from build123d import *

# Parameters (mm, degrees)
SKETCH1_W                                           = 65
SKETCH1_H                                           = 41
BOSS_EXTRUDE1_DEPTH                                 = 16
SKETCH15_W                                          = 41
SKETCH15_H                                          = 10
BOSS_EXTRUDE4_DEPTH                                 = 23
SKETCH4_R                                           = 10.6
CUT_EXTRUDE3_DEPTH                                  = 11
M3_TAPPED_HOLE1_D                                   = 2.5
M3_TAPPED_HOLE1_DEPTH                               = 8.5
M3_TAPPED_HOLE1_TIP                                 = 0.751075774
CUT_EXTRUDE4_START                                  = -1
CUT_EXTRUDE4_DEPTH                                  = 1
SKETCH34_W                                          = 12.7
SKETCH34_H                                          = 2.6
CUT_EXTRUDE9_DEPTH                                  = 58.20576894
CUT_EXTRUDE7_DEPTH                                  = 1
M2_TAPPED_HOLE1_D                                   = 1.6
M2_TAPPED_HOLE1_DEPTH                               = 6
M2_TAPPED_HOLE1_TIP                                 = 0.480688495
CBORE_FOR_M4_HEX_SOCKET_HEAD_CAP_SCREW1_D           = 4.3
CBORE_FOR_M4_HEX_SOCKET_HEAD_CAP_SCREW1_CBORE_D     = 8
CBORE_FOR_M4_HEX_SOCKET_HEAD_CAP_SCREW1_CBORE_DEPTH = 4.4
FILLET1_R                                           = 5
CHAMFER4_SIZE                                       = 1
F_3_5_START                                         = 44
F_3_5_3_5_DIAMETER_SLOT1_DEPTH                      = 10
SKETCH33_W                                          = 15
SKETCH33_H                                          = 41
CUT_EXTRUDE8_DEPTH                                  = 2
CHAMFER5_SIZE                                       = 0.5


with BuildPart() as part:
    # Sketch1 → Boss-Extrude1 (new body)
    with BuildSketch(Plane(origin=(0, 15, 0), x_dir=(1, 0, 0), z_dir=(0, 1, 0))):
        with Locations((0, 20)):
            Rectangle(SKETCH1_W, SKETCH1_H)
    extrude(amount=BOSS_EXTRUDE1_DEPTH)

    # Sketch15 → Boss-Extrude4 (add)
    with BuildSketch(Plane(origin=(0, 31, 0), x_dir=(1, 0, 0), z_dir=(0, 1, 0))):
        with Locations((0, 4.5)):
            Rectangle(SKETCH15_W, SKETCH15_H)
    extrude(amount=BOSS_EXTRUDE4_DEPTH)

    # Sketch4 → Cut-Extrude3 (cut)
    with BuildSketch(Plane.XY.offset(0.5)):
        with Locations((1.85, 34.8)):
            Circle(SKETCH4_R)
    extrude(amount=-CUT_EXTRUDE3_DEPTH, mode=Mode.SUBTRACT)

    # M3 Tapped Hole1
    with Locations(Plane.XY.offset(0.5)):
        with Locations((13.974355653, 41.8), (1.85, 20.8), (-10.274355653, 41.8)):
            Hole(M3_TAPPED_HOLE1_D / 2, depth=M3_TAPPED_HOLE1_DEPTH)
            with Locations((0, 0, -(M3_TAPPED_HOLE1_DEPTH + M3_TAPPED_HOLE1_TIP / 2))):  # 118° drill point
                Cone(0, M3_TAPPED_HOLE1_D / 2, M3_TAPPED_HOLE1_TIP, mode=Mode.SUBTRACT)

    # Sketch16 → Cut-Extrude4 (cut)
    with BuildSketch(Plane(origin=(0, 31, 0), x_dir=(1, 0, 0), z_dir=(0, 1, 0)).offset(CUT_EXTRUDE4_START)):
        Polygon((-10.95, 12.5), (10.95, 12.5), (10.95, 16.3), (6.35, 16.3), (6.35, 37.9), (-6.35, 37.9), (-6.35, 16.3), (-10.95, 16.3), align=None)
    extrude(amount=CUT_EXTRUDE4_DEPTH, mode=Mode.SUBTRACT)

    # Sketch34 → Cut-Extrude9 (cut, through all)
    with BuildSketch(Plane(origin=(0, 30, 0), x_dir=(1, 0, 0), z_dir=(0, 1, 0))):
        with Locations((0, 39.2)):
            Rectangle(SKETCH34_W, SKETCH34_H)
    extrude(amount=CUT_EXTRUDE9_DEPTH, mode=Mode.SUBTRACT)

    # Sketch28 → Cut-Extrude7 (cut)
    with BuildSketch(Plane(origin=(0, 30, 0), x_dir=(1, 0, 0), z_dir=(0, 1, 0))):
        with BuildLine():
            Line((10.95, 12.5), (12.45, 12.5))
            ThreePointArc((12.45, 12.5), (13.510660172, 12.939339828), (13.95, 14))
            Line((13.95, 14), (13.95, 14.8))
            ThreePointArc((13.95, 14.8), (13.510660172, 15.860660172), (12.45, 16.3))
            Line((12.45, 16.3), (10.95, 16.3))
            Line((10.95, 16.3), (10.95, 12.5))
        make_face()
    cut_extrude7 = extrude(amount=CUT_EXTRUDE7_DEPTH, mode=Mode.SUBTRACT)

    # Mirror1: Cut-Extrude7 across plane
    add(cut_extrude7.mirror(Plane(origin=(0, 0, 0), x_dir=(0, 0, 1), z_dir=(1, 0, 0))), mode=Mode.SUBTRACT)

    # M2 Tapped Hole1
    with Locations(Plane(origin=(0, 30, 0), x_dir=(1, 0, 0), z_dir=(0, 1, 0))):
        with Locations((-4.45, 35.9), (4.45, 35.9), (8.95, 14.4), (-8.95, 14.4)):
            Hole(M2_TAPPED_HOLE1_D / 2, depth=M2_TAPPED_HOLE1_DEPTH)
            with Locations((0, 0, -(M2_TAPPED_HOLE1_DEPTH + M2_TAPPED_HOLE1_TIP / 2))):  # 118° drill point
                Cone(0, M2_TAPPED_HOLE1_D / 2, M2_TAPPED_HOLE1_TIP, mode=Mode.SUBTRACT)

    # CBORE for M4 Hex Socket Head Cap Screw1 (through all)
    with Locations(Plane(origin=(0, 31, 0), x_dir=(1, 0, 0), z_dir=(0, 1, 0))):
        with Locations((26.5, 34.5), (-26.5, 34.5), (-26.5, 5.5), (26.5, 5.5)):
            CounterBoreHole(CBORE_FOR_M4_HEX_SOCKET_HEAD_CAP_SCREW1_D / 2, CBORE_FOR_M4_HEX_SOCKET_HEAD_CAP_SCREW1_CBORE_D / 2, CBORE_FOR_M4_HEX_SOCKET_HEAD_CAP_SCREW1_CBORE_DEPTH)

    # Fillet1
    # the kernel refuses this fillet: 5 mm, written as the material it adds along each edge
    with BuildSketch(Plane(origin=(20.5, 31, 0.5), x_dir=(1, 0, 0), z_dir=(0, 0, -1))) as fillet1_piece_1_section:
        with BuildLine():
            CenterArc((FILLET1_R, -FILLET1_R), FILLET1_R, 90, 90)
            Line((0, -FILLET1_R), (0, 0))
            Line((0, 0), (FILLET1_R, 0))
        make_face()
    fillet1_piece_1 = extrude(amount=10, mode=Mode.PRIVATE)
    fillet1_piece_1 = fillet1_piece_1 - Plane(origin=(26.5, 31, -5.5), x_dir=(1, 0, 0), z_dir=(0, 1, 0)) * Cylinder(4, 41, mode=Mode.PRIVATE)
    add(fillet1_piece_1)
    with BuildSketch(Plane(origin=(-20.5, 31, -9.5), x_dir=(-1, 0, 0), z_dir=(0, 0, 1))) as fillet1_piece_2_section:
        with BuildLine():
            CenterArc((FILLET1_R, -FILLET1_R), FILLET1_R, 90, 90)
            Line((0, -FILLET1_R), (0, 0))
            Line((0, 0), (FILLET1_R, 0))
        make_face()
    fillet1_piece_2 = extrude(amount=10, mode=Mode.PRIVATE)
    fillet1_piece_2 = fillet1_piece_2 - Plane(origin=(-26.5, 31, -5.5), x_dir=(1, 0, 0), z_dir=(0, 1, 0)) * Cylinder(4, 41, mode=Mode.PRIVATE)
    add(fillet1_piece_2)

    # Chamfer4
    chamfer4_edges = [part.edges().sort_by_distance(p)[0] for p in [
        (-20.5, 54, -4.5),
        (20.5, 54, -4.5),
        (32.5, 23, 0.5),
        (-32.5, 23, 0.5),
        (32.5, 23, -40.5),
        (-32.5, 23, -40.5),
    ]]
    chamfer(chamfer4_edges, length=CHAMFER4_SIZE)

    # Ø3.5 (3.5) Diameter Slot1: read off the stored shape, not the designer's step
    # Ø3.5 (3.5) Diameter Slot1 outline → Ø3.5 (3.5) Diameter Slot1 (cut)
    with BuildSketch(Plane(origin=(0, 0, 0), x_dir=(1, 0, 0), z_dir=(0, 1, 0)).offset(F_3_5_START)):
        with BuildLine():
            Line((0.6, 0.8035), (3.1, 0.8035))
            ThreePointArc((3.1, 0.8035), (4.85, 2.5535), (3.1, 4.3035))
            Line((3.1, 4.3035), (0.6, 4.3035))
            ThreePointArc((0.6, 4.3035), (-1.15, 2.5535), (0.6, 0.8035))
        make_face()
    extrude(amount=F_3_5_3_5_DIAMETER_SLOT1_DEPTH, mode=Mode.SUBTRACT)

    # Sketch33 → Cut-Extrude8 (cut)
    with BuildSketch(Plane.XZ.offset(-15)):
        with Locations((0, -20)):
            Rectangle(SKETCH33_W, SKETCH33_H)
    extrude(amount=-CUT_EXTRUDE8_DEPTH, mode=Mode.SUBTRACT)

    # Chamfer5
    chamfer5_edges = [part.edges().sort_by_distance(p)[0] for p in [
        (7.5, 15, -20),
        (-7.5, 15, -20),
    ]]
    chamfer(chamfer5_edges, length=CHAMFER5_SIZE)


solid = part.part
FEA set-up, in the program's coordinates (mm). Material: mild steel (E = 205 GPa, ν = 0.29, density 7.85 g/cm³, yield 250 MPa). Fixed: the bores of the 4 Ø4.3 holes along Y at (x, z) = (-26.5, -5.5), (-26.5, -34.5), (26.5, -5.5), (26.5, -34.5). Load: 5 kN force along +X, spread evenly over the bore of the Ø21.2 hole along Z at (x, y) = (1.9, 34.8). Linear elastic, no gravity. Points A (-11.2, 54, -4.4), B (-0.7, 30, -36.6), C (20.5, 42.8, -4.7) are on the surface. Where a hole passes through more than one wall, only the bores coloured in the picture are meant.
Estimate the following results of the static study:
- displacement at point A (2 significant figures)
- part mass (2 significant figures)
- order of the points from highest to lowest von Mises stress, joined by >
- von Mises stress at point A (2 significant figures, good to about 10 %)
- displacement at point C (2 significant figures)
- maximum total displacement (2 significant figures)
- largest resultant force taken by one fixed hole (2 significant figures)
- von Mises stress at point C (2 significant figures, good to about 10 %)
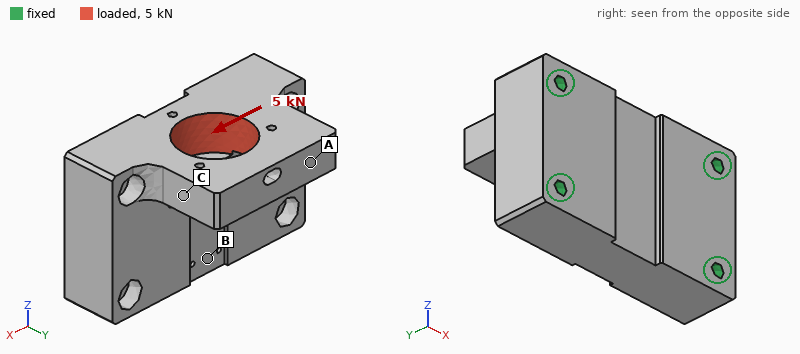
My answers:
6.6 µm
350 g
C > A > B
12 MPa
5.6 µm
6.8 µm
2.3 kN
20 MPa
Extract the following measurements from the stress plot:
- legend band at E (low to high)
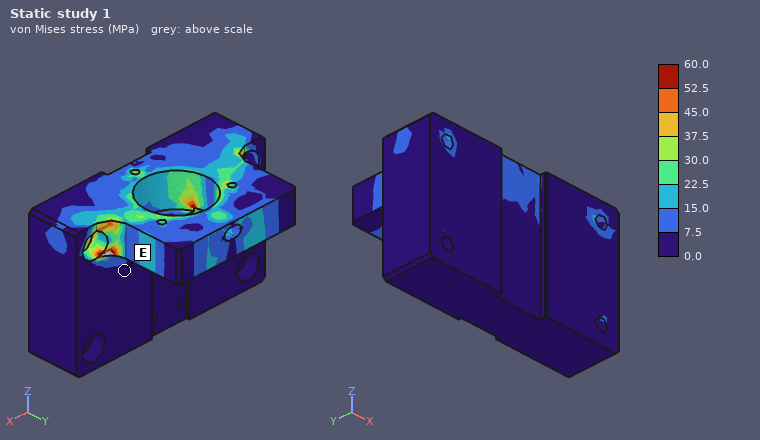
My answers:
0.0 to 7.5 MPa
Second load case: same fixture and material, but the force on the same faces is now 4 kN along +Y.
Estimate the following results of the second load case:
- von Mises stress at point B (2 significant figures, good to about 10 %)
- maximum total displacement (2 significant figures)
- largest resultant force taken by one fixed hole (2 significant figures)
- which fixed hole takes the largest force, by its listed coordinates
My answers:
4.0 MPa
4.5 µm
2.2 kN
(26.5, -5.5)
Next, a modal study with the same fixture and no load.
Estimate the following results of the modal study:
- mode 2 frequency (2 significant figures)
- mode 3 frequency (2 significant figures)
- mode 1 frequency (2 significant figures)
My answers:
13 kHz
15 kHz
7500 Hz
